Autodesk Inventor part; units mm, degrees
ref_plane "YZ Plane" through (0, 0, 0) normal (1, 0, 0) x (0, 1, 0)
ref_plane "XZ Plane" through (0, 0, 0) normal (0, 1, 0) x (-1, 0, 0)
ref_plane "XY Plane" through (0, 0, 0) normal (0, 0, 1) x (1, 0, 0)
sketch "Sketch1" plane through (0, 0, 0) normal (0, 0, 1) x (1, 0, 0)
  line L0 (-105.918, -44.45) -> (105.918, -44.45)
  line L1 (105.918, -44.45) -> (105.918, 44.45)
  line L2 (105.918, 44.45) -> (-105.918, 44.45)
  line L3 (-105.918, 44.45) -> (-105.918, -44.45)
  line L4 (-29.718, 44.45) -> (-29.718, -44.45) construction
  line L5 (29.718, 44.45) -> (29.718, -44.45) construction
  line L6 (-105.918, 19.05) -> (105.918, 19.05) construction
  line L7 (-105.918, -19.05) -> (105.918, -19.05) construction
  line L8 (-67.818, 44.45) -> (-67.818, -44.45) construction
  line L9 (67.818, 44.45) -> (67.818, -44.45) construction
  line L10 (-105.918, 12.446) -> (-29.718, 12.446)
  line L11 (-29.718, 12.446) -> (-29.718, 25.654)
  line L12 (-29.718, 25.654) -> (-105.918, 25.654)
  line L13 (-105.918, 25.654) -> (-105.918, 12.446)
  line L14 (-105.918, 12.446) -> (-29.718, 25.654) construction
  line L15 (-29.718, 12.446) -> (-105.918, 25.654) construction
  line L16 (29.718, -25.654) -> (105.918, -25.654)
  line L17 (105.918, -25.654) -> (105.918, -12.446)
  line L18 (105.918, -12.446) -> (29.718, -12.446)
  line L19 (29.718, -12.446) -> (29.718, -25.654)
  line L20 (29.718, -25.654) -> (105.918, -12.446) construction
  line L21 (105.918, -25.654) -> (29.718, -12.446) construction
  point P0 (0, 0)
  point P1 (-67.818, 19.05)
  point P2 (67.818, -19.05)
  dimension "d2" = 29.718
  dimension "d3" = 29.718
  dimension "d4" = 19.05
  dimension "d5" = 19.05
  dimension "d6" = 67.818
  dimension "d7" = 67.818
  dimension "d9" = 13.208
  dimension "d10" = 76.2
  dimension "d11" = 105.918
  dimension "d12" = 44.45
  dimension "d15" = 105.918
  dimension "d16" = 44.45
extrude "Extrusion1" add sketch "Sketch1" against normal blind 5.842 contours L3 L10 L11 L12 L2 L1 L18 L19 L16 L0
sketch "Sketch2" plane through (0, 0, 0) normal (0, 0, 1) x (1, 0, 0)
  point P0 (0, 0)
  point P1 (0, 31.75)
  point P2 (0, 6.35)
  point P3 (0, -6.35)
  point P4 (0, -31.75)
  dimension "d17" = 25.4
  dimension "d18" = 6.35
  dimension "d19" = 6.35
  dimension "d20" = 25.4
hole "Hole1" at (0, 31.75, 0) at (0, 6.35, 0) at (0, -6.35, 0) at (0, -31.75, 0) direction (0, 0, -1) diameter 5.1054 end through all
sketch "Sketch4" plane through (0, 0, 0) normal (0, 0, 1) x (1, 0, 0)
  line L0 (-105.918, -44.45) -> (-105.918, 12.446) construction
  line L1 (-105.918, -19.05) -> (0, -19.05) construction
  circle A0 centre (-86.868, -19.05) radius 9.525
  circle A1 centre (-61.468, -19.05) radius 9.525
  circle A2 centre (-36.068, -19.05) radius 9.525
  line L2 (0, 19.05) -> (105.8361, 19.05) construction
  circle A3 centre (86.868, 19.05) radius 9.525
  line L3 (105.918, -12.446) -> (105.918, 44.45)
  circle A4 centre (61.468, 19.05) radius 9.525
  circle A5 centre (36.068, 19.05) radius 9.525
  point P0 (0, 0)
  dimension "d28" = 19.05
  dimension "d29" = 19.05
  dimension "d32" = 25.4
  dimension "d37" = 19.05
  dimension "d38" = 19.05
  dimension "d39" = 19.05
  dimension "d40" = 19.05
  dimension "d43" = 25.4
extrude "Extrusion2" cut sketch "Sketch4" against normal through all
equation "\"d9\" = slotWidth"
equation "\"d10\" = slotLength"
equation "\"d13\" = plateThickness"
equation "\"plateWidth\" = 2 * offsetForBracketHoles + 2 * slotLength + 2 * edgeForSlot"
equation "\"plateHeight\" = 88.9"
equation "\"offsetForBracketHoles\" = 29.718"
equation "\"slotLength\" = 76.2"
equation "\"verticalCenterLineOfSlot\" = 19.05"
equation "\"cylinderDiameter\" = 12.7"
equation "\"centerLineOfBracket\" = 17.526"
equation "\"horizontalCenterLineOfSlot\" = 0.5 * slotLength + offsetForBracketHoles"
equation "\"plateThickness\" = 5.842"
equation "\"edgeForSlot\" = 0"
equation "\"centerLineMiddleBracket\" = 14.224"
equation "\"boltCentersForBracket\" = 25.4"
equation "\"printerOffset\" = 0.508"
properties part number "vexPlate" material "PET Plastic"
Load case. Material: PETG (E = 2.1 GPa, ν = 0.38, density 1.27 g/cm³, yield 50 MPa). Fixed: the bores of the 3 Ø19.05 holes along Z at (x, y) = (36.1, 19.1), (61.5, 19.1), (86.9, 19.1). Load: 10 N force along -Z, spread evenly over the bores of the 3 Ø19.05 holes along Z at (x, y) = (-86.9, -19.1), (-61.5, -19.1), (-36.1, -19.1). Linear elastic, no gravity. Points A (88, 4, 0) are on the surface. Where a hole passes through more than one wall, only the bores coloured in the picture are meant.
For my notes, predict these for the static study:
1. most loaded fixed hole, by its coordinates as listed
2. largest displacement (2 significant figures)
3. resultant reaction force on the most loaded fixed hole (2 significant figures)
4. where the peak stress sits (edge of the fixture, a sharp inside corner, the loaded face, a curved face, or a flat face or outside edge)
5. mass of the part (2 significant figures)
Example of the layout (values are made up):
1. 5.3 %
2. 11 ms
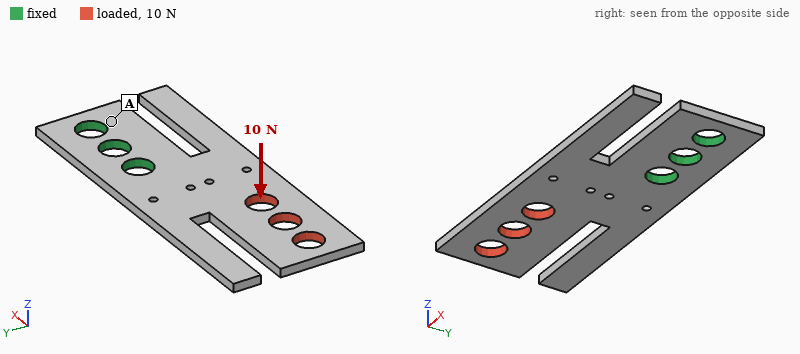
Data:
1. (36.1, 19.1)
2. 2.6 mm
3. 15 N
4. a flat face or outside edge
5. 110 g
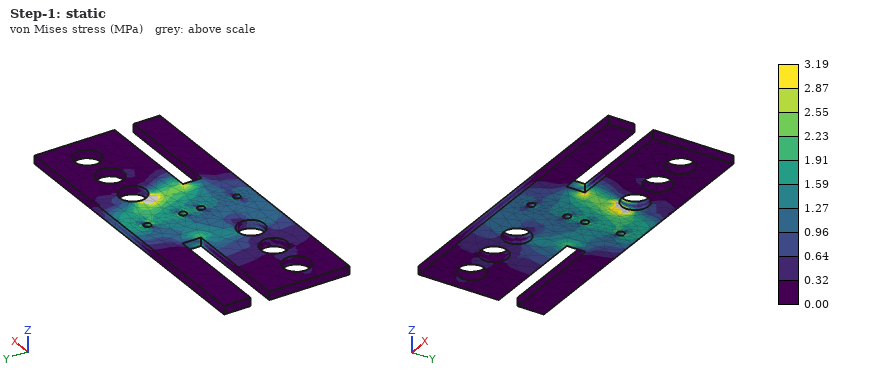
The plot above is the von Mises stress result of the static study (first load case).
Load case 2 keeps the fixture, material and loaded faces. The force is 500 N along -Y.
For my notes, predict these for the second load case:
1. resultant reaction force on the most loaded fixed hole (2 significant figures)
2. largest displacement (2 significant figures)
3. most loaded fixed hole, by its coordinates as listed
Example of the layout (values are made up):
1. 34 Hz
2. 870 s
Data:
1. 1.1 kN
2. 2.3 mm
3. (36.1, 19.1)
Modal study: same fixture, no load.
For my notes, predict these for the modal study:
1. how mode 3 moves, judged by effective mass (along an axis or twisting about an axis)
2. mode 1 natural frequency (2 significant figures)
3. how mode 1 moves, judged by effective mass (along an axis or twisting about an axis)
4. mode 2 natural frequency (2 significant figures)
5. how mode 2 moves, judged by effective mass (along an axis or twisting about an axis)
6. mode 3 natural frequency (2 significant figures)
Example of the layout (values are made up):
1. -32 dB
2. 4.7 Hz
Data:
1. along Z
2. 65 Hz
3. along Z
4. 120 Hz
5. twisting about X
6. 130 Hz
